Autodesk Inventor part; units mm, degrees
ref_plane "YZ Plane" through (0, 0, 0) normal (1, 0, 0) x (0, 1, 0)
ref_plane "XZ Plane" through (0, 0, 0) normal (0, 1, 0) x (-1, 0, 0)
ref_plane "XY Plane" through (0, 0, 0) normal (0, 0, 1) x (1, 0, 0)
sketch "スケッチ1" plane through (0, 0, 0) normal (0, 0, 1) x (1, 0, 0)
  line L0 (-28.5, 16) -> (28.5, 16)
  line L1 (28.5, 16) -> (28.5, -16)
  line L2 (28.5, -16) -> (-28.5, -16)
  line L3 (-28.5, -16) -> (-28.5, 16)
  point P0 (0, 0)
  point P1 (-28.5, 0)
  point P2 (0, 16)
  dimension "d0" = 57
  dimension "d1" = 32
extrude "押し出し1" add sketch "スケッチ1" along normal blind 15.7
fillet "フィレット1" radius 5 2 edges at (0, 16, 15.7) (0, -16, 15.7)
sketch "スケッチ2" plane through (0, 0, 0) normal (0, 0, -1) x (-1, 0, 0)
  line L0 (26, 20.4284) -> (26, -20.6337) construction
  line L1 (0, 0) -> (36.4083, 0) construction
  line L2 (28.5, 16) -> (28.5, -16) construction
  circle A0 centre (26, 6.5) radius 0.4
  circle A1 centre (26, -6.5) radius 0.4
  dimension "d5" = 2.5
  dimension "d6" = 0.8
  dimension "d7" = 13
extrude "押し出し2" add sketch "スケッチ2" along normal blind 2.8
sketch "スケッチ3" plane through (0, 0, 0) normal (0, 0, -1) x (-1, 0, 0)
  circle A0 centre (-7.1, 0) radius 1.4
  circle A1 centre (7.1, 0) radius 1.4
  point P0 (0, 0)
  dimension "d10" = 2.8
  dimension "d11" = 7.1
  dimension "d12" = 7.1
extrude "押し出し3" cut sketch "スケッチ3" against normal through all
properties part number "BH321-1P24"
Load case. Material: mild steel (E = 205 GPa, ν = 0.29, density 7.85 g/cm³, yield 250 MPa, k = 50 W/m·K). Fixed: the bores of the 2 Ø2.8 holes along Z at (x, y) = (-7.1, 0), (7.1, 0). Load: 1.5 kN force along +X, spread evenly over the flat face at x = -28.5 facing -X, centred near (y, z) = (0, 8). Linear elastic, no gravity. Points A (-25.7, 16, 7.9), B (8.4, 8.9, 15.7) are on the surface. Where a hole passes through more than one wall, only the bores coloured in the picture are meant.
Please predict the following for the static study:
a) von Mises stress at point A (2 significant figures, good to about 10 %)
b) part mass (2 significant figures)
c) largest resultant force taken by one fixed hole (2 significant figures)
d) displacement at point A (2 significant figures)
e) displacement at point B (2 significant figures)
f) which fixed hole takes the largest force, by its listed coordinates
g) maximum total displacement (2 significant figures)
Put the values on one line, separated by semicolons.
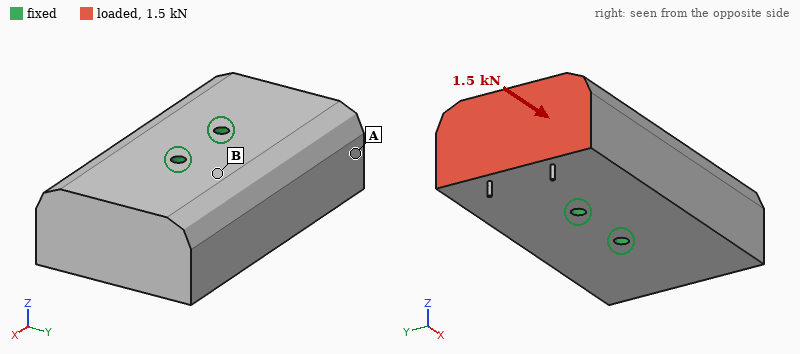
3.0 MPa; 220 g; 1.0 kN; 0.45 µm; 0.095 µm; (-7.1, 0); 0.50 µm
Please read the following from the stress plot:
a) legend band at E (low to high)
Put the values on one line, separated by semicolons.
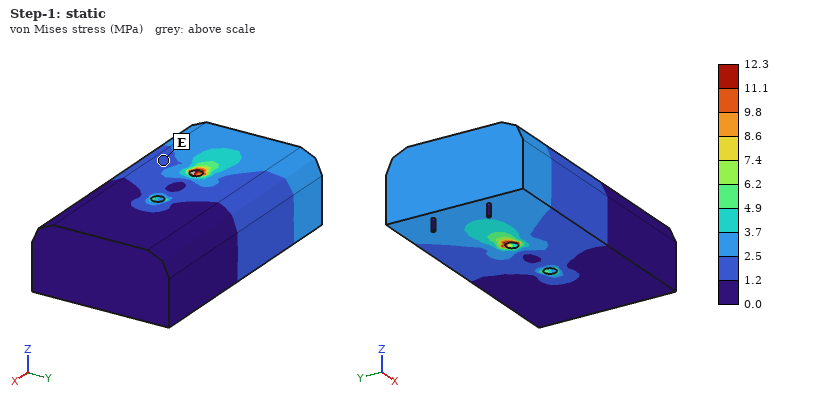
1.2 to 2.5 MPa
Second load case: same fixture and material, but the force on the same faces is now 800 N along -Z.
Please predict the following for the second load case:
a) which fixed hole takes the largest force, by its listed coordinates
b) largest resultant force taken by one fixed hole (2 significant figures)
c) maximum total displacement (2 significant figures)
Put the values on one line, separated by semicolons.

(-7.1, 0); 1.1 kN; 3.1 µm
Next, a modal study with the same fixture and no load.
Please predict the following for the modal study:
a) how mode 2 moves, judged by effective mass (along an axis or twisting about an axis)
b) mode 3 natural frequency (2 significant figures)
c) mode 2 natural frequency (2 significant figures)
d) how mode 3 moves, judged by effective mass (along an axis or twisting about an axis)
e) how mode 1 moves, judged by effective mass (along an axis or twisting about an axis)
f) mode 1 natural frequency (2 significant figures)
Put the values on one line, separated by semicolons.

twisting about Y; 17 kHz; 14 kHz; along Z; twisting about Z; 13 kHz
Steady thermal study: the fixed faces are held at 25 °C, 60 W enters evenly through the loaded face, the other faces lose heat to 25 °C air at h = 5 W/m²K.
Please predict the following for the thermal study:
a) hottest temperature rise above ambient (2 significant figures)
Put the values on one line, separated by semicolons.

64 K
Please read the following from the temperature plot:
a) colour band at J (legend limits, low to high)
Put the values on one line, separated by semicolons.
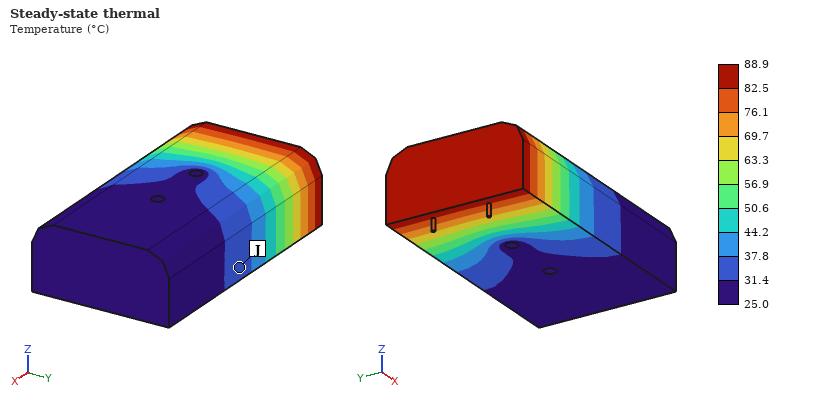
31.4 to 37.8 °C
